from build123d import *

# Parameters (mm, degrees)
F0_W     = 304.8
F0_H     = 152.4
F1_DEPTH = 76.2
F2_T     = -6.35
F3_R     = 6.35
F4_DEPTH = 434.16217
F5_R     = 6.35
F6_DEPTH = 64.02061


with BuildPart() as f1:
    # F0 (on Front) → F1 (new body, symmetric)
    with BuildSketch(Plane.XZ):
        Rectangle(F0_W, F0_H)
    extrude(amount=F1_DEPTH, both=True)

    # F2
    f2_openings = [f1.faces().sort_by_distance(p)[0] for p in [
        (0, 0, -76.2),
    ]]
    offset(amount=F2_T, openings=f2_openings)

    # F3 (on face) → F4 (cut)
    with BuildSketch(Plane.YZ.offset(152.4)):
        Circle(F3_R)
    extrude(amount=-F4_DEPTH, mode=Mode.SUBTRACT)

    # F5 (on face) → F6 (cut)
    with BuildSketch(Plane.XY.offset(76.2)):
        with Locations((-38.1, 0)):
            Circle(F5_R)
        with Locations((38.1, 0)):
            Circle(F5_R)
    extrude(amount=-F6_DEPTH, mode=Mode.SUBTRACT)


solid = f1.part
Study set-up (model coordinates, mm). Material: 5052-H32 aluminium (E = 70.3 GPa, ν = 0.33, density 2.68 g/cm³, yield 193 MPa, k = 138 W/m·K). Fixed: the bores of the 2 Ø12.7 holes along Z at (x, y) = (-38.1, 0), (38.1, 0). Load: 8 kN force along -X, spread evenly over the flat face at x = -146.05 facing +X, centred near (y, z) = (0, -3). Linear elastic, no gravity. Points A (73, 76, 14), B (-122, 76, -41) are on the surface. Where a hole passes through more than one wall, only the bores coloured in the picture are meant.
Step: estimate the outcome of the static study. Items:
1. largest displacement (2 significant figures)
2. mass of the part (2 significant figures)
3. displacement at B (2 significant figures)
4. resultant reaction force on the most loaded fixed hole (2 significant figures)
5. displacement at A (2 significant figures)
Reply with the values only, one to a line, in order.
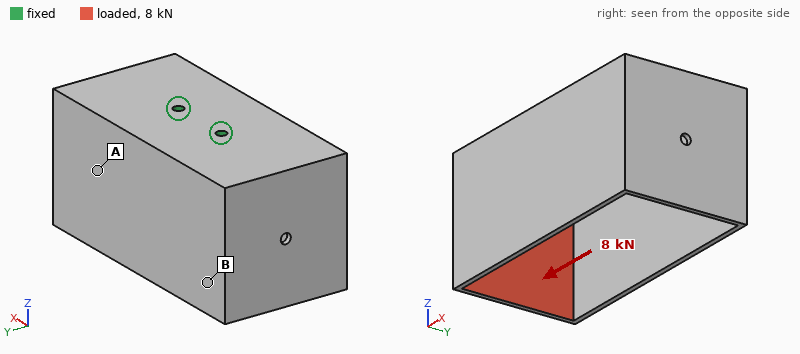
3.2 mm
3.0 kg
2.0 mm
7.1 kN
1.2 mm
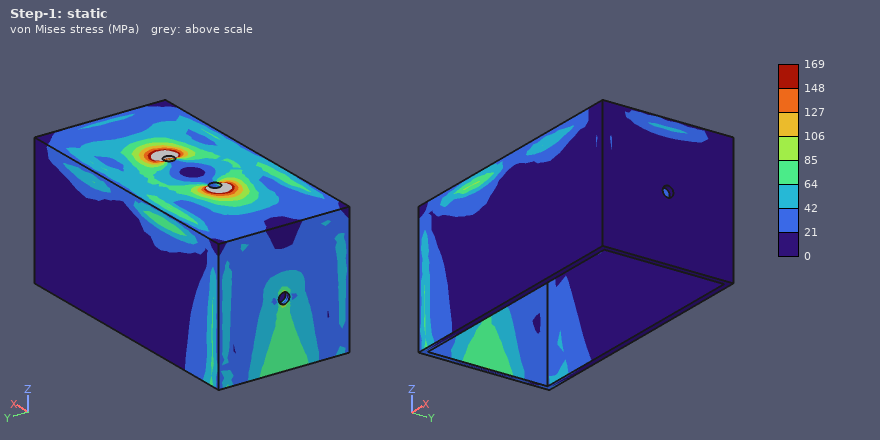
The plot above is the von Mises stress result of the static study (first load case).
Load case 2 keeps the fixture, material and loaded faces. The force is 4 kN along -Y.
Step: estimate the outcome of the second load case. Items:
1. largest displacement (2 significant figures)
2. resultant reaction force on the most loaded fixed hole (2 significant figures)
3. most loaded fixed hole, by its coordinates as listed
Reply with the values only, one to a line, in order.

3.8 mm
9.0 kN
(-38.1, 0)
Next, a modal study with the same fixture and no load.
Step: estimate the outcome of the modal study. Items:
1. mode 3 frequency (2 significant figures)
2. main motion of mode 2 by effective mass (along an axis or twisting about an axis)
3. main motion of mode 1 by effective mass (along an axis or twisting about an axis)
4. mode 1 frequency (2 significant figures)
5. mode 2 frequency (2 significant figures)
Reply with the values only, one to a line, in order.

240 Hz
along X
along Y
130 Hz
160 Hz
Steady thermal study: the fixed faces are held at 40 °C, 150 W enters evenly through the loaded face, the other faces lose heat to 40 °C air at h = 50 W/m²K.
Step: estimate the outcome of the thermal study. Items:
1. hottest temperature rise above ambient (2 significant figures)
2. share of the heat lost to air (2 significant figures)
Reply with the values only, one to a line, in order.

41 K
88 %
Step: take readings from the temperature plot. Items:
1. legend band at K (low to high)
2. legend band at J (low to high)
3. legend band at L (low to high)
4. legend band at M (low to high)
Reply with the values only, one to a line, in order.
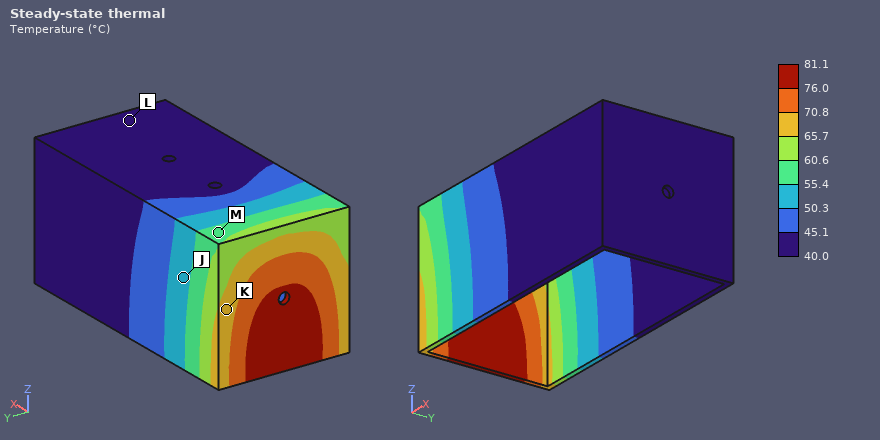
65.7 to 70.8 °C
50.3 to 55.4 °C
40.0 to 45.1 °C
55.4 to 60.6 °C
